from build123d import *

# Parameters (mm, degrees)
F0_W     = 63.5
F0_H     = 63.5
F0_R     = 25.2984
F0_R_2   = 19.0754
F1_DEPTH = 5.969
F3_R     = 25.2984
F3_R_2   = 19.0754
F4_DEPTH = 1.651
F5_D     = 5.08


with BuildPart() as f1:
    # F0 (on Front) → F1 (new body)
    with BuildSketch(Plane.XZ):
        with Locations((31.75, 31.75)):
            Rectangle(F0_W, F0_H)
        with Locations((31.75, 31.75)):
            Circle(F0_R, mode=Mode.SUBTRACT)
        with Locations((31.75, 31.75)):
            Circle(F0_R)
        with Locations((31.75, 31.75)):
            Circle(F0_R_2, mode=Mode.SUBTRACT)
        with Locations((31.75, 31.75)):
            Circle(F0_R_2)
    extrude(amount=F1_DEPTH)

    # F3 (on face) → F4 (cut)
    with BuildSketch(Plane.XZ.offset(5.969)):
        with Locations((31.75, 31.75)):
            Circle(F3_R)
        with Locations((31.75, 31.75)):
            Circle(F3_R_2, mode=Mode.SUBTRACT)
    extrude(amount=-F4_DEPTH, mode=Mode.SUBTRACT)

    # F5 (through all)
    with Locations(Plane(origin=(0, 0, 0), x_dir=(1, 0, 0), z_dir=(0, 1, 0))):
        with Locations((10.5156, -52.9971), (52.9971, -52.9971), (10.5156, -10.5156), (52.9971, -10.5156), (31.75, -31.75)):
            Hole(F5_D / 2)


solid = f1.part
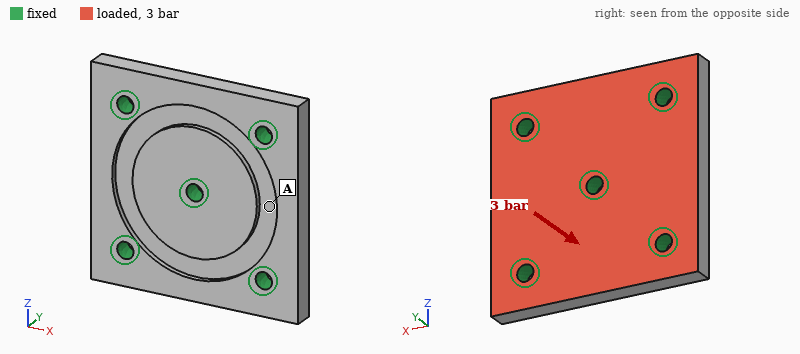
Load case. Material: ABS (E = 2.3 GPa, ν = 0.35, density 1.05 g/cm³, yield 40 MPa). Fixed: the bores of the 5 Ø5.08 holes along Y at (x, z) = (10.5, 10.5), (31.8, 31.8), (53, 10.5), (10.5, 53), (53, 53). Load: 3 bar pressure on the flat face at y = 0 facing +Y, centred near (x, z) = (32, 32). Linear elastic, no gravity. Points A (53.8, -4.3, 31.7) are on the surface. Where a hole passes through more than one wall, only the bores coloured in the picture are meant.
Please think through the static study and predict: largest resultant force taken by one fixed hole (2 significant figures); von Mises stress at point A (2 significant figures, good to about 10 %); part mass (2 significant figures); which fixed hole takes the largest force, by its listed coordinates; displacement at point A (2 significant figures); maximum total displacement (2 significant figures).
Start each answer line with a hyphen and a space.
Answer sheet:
- 280 N
- 1.7 MPa
- 23 g
- (31.8, 31.8)
- 58 µm
- 83 µm
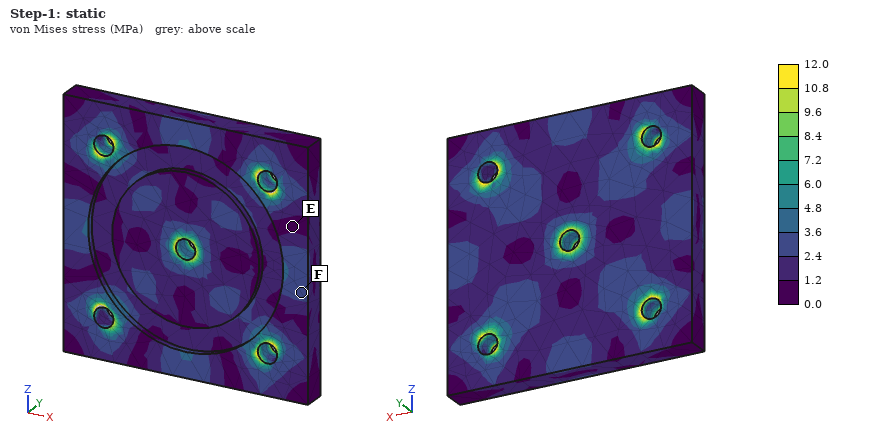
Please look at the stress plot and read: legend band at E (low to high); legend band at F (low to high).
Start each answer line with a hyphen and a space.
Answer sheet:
- 0.0 to 1.2 MPa
- 2.4 to 3.6 MPa
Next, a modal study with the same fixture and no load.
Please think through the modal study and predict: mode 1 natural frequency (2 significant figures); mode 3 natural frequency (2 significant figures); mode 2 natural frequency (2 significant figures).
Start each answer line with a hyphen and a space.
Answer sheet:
- 4700 Hz
- 4900 Hz
- 4900 Hz
